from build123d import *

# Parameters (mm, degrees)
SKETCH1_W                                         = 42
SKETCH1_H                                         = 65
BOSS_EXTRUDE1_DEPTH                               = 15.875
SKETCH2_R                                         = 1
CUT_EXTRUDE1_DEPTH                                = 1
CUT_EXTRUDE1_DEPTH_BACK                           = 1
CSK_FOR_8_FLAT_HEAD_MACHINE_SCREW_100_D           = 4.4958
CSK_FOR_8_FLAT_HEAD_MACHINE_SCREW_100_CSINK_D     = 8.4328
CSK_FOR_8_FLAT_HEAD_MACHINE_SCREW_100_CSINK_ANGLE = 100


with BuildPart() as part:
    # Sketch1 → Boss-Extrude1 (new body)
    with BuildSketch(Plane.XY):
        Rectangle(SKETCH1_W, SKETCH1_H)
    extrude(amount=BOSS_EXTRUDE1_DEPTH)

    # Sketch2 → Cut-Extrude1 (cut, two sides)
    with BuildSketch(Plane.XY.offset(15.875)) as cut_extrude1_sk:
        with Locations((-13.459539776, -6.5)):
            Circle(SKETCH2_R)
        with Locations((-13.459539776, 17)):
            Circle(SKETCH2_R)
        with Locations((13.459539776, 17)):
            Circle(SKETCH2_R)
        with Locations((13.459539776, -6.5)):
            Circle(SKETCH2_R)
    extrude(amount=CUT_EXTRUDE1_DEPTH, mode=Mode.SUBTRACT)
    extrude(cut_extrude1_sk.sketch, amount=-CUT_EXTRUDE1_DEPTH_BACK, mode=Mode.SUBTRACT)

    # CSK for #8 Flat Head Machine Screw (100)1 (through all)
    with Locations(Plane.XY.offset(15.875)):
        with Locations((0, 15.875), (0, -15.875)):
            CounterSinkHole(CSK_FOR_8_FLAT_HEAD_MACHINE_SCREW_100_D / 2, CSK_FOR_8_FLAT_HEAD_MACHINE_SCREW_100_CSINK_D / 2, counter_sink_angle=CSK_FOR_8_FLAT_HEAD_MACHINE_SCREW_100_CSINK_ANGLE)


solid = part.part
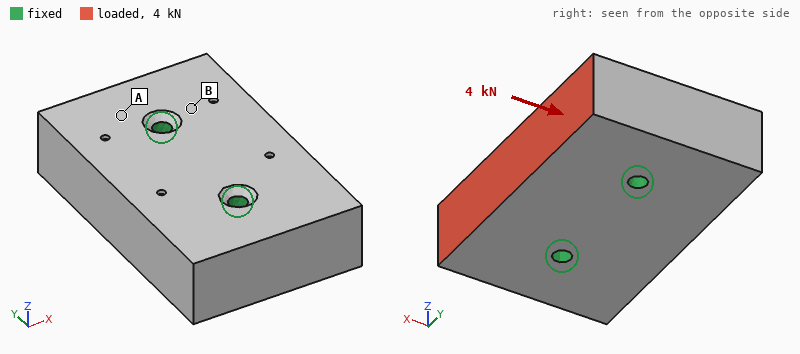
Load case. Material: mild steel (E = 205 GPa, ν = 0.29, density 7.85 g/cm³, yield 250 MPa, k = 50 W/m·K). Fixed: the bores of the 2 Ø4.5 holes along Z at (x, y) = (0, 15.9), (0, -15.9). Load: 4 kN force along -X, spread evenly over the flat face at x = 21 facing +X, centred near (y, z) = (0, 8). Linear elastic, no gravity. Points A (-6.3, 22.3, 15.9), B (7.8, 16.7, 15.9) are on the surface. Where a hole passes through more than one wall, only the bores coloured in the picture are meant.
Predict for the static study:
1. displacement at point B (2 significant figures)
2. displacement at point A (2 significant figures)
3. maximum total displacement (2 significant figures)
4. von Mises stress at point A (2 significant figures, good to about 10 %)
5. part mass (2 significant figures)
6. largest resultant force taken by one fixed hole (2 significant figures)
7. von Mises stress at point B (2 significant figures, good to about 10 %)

0.33 µm
0.26 µm
0.87 µm
2.6 MPa
340 g
2.0 kN
5.5 MPa
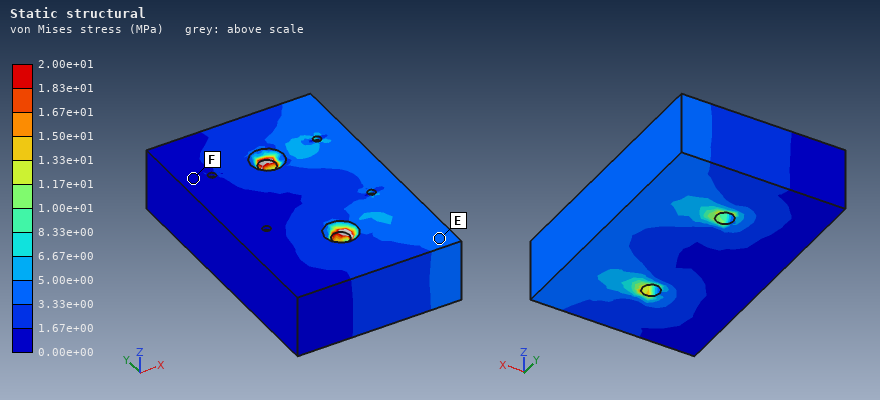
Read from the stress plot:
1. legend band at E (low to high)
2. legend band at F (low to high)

3.33e+00 to 5.00e+00 MPa
0.00e+00 to 1.67e+00 MPa
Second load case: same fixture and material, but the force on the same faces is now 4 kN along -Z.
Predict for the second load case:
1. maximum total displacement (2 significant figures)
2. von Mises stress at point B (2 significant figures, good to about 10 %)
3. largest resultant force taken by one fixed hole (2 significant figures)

7.6 µm
21 MPa
2.0 kN
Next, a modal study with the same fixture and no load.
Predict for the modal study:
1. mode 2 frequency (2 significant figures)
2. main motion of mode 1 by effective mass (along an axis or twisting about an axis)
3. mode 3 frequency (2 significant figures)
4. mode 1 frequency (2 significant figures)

19 kHz
twisting about Y
19 kHz
13 kHz
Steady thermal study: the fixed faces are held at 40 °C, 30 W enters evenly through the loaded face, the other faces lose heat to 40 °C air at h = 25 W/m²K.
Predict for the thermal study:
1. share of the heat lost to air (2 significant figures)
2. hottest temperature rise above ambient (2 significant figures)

3.5 %
15 K
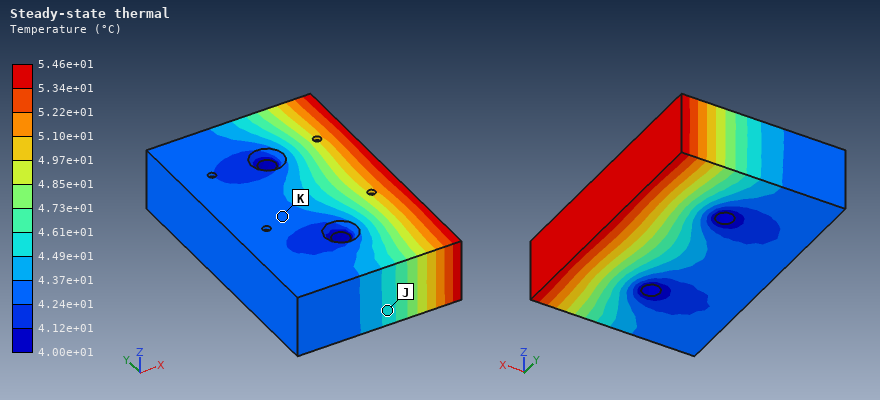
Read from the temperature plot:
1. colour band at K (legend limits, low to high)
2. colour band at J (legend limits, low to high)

4.24e+01 to 4.37e+01 °C
4.49e+01 to 4.61e+01 °C
